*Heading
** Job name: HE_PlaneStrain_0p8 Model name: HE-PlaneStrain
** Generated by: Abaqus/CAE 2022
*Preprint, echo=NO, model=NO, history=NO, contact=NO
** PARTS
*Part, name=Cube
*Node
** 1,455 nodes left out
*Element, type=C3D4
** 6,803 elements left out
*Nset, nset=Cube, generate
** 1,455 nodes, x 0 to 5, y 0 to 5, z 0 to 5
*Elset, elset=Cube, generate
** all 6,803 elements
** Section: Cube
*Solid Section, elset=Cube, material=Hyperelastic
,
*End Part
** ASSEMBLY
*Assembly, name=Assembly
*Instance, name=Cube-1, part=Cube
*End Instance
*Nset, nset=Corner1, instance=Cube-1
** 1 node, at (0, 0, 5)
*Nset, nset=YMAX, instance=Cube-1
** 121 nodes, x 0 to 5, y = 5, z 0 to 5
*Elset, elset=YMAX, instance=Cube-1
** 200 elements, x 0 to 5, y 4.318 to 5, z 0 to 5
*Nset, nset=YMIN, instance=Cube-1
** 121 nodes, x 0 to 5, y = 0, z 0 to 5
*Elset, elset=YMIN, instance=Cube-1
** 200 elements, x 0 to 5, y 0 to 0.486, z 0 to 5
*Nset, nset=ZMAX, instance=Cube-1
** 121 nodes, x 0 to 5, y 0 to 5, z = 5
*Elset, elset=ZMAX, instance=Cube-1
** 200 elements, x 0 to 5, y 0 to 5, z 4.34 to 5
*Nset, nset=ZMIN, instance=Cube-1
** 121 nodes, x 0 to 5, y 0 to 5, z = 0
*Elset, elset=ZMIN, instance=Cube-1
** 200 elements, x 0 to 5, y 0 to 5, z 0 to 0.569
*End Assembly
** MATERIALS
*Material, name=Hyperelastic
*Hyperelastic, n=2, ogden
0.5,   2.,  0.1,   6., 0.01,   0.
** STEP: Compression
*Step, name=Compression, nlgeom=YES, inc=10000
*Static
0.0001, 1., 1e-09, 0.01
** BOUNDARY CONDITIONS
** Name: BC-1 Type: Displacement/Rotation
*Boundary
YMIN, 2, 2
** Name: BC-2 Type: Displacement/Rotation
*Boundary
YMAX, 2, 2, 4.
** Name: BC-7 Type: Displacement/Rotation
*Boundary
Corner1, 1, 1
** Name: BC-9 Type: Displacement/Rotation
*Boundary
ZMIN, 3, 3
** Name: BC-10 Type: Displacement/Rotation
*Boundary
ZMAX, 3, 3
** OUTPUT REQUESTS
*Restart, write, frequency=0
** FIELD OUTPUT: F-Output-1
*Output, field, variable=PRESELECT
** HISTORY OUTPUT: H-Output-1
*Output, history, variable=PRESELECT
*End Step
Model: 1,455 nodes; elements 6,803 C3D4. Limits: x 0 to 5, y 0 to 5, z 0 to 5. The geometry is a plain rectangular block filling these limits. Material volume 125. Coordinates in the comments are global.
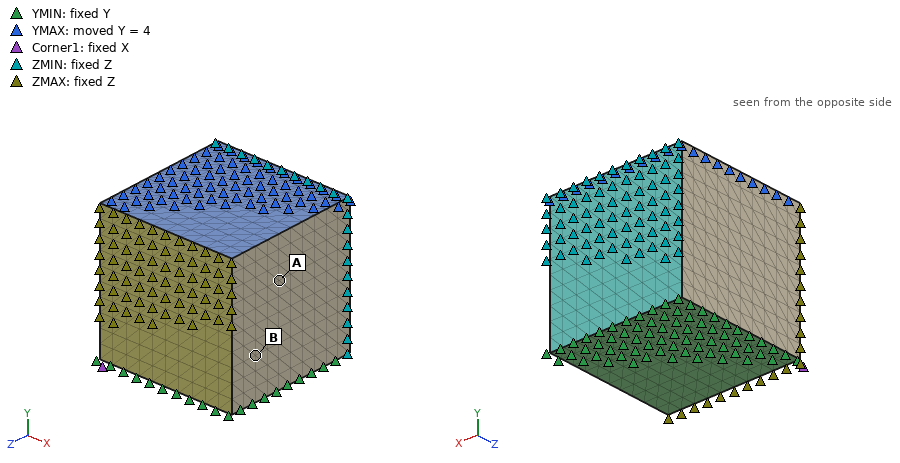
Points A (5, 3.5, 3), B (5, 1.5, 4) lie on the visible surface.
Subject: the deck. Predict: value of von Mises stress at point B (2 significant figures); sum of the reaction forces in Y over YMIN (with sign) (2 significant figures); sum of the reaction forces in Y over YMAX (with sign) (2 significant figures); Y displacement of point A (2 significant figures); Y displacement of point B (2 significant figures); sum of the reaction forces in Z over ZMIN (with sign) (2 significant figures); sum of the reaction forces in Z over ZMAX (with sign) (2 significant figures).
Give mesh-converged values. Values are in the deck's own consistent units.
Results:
1.3
-20
20
2.8
1.2
-8.3
8.3
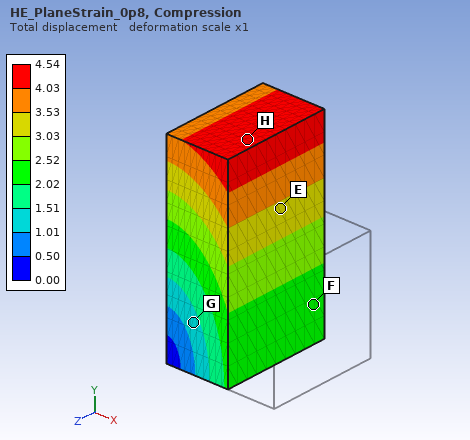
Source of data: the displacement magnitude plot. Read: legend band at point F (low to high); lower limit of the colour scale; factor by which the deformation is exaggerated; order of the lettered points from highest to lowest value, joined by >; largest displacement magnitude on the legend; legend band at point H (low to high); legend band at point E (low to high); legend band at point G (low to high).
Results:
2.02 to 2.52
0.00
1
H > E > F > G
4.54
4.03 to 4.54
3.03 to 3.53
1.01 to 1.51
